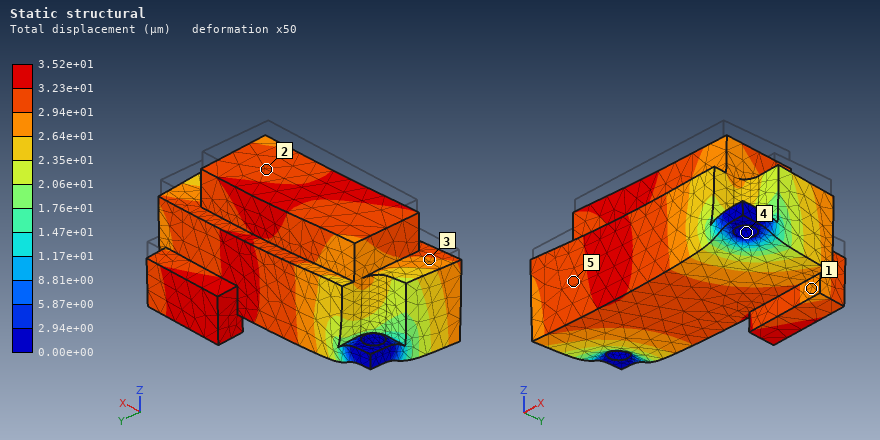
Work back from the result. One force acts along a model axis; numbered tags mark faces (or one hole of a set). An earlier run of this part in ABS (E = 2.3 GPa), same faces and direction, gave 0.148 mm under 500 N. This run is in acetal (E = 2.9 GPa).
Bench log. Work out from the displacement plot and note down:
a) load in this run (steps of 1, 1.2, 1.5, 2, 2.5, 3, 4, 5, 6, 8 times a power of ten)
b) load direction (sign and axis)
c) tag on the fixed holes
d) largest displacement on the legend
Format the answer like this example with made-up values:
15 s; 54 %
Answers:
150 N; -Z; 4; 3.52e+01 µm
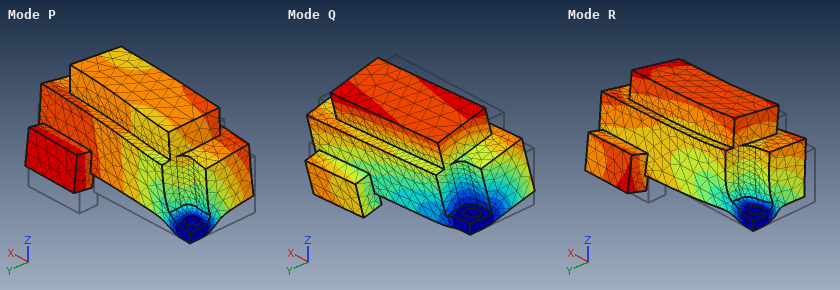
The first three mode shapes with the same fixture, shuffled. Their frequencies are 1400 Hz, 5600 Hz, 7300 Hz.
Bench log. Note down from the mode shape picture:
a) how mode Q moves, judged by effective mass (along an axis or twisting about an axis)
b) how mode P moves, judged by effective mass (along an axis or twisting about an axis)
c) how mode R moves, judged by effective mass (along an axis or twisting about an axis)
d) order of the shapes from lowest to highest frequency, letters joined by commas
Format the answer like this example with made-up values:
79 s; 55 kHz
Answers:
along Y; along Z; along X; Q, P, R
